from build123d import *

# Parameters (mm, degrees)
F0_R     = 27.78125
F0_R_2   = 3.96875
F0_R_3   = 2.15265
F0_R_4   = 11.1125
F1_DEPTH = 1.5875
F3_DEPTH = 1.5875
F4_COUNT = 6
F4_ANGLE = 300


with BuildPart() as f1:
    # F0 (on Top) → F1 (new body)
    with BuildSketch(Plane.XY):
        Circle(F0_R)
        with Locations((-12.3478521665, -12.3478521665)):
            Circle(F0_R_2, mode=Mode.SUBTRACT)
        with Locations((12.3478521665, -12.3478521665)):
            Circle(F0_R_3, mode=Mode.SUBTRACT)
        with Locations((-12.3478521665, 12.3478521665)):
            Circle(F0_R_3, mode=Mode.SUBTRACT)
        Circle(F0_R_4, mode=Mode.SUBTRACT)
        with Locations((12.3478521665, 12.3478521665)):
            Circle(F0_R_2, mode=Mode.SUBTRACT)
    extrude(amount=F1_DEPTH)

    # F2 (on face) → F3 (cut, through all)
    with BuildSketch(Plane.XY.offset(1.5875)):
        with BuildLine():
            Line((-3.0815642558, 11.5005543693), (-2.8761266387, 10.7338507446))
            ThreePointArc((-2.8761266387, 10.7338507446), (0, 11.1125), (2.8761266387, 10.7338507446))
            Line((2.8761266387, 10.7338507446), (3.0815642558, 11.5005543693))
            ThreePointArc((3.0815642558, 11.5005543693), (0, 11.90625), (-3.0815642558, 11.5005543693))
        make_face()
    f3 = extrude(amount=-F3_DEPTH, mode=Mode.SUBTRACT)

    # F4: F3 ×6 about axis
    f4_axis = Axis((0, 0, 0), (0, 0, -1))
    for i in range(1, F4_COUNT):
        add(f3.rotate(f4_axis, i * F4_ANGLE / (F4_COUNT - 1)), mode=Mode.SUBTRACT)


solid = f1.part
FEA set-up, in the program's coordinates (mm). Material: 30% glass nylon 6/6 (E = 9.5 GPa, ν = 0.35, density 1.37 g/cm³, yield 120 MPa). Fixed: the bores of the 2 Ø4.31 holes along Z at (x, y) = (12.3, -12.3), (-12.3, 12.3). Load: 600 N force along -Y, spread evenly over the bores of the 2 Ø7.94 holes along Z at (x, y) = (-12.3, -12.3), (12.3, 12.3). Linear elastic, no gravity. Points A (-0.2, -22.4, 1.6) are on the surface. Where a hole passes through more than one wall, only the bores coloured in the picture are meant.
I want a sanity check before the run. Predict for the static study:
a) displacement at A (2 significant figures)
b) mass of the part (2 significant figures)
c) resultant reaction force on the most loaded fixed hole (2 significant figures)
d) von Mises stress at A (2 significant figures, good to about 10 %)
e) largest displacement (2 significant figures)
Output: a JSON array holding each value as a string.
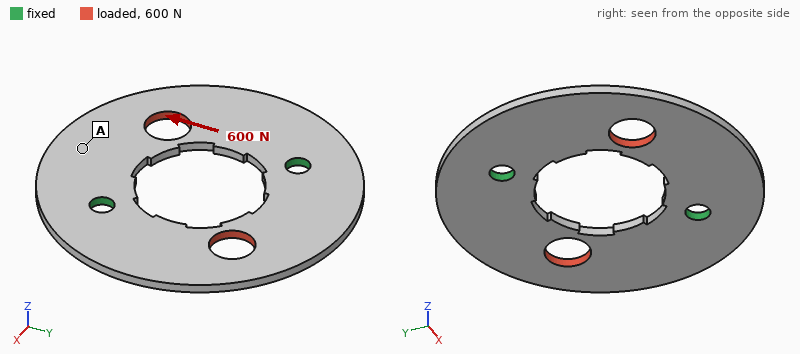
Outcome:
["31 µm", "4.1 g", "300 N", "5.8 MPa", "54 µm"]
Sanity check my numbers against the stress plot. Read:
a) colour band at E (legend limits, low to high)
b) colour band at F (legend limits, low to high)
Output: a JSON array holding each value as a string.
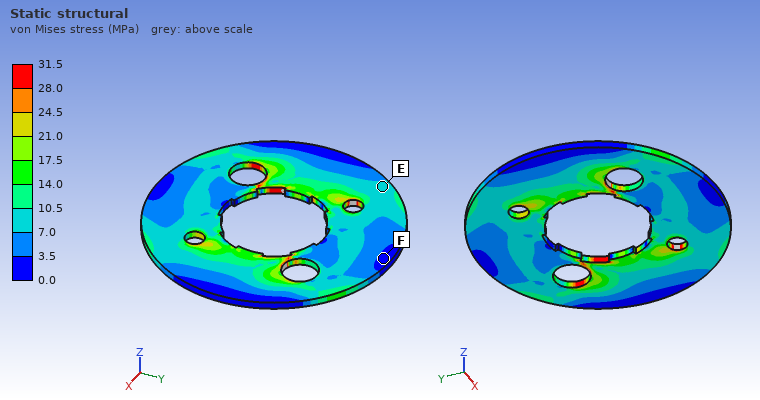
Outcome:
["7.0 to 10.5 MPa", "0.0 to 3.5 MPa"]
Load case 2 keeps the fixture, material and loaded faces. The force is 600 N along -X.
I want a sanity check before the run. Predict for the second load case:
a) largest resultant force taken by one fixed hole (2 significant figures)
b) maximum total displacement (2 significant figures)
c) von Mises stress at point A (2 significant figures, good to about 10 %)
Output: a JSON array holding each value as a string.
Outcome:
["300 N", "55 µm", "5.0 MPa"]
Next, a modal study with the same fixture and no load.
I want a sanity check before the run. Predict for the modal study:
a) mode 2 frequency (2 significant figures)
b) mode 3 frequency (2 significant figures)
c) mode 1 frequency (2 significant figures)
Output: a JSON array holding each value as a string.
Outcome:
["980 Hz", "2200 Hz", "970 Hz"]
